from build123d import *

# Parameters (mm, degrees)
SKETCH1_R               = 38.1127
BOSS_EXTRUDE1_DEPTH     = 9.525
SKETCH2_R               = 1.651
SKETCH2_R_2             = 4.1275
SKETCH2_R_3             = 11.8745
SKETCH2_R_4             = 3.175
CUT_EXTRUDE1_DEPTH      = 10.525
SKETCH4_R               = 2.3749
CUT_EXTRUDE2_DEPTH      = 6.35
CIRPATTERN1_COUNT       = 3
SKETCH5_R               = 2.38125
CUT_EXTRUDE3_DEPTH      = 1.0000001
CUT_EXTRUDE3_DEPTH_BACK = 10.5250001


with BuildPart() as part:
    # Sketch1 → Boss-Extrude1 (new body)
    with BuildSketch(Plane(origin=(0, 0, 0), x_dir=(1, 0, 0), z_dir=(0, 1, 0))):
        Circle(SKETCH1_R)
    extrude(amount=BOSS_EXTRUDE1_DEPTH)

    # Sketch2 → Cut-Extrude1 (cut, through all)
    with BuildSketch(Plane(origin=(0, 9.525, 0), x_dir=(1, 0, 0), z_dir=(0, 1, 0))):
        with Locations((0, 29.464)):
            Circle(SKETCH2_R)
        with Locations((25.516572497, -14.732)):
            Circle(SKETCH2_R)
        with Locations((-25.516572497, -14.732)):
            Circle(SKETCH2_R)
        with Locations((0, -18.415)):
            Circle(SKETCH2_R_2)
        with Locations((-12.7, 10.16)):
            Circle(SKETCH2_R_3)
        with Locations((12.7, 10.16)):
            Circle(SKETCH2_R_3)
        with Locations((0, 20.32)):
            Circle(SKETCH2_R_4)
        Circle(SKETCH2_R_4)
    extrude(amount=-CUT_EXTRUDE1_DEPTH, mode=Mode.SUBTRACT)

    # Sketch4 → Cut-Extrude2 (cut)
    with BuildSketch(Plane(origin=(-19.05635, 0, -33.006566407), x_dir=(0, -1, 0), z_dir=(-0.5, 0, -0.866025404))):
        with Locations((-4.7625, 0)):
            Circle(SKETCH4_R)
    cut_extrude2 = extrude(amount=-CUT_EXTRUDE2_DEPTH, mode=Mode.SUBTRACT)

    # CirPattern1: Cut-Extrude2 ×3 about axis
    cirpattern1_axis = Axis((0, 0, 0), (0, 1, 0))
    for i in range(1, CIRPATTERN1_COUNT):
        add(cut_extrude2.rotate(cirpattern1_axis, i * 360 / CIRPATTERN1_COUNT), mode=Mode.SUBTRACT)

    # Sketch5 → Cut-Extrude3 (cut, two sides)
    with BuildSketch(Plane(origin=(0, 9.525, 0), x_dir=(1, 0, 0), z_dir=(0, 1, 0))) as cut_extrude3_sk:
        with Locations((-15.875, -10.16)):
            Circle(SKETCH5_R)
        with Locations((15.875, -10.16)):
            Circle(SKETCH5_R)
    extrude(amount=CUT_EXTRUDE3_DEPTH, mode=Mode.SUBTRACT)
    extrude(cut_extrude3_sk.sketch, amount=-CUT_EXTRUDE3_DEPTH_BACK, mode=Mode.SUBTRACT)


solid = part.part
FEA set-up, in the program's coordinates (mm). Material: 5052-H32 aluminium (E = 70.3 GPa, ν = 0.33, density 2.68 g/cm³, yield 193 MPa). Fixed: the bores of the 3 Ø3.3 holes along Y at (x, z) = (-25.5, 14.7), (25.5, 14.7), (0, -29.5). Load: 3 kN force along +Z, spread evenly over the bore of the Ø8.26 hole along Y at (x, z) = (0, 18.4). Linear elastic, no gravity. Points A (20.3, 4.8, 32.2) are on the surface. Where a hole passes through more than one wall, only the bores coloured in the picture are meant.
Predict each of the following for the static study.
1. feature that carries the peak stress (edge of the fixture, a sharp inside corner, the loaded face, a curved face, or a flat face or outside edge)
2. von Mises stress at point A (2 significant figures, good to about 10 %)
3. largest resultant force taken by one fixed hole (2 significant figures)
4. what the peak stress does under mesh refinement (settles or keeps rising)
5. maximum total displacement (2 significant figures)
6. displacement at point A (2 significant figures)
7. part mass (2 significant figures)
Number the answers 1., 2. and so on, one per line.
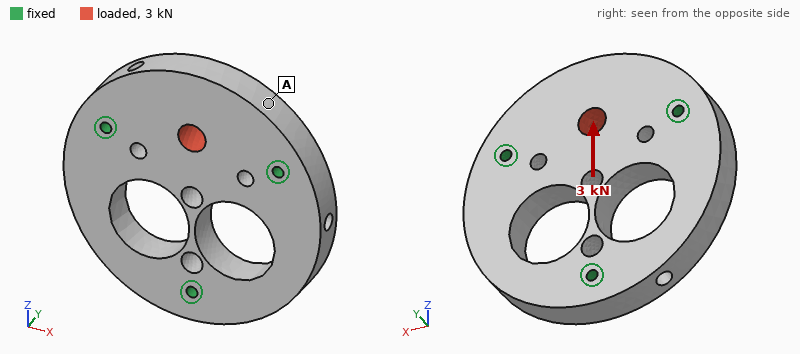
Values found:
1. edge of the fixture
2. 7.1 MPa
3. 1.5 kN
4. keeps rising
5. 8.0 µm
6. 3.3 µm
7. 88 g
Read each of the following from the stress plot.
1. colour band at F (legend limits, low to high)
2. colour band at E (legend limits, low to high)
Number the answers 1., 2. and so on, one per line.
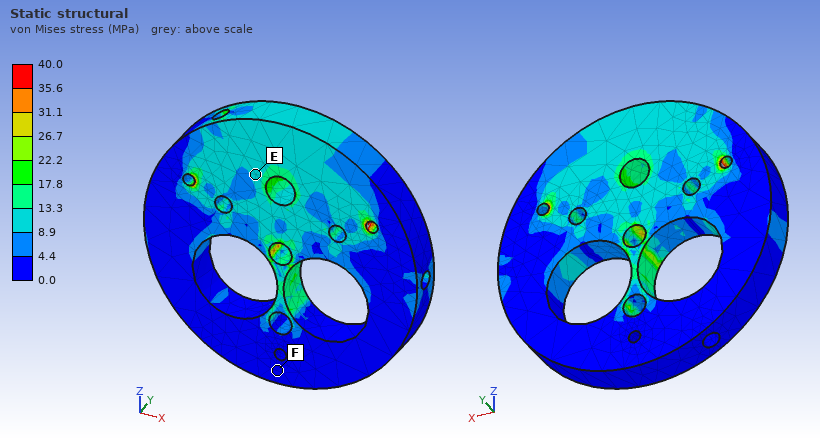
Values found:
1. 0.0 to 4.4 MPa
2. 8.9 to 13.3 MPa
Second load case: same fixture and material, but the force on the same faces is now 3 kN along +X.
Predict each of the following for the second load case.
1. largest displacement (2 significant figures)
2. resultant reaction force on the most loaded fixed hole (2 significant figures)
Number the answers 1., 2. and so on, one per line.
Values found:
1. 4.2 µm
2. 1.5 kN
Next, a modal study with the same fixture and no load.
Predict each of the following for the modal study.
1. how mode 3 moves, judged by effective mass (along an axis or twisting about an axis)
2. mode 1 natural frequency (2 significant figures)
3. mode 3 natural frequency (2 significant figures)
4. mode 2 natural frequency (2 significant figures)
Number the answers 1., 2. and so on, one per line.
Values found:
1. along Y
2. 8600 Hz
3. 10 kHz
4. 9000 Hz
